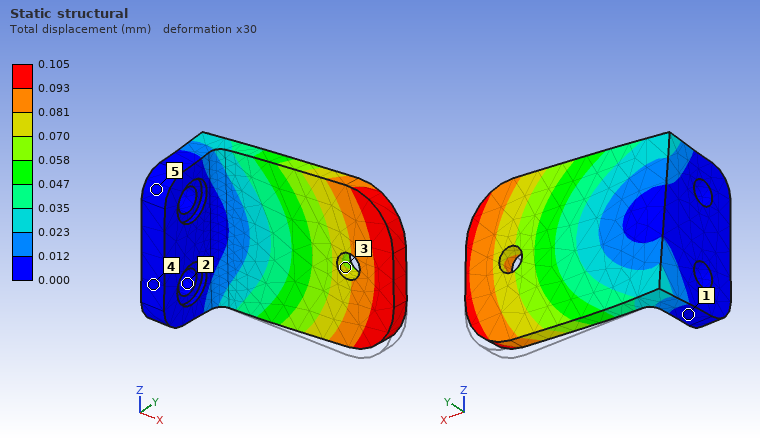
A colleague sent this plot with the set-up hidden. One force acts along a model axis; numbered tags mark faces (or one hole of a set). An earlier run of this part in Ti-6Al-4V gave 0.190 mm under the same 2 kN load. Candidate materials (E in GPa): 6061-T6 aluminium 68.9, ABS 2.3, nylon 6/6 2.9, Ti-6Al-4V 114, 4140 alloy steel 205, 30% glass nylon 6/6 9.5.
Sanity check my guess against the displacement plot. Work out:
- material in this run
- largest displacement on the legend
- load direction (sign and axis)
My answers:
4140 alloy steel
0.105 mm
+Z
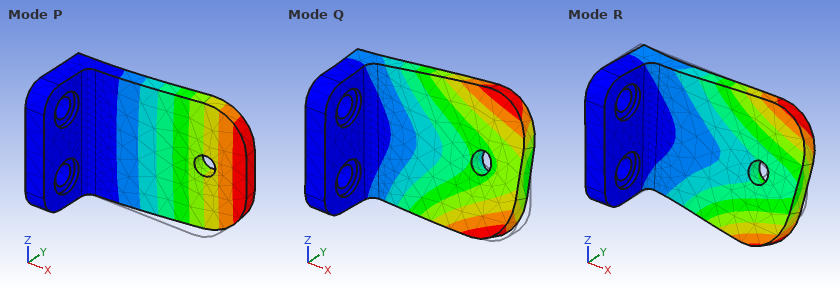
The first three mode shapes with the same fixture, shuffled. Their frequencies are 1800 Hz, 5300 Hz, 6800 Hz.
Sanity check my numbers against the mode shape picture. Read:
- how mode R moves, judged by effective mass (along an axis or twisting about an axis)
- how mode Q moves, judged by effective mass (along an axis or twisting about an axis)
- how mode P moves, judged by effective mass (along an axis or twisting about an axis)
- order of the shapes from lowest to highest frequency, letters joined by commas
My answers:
along Z
along Z
along Y
P, Q, R
